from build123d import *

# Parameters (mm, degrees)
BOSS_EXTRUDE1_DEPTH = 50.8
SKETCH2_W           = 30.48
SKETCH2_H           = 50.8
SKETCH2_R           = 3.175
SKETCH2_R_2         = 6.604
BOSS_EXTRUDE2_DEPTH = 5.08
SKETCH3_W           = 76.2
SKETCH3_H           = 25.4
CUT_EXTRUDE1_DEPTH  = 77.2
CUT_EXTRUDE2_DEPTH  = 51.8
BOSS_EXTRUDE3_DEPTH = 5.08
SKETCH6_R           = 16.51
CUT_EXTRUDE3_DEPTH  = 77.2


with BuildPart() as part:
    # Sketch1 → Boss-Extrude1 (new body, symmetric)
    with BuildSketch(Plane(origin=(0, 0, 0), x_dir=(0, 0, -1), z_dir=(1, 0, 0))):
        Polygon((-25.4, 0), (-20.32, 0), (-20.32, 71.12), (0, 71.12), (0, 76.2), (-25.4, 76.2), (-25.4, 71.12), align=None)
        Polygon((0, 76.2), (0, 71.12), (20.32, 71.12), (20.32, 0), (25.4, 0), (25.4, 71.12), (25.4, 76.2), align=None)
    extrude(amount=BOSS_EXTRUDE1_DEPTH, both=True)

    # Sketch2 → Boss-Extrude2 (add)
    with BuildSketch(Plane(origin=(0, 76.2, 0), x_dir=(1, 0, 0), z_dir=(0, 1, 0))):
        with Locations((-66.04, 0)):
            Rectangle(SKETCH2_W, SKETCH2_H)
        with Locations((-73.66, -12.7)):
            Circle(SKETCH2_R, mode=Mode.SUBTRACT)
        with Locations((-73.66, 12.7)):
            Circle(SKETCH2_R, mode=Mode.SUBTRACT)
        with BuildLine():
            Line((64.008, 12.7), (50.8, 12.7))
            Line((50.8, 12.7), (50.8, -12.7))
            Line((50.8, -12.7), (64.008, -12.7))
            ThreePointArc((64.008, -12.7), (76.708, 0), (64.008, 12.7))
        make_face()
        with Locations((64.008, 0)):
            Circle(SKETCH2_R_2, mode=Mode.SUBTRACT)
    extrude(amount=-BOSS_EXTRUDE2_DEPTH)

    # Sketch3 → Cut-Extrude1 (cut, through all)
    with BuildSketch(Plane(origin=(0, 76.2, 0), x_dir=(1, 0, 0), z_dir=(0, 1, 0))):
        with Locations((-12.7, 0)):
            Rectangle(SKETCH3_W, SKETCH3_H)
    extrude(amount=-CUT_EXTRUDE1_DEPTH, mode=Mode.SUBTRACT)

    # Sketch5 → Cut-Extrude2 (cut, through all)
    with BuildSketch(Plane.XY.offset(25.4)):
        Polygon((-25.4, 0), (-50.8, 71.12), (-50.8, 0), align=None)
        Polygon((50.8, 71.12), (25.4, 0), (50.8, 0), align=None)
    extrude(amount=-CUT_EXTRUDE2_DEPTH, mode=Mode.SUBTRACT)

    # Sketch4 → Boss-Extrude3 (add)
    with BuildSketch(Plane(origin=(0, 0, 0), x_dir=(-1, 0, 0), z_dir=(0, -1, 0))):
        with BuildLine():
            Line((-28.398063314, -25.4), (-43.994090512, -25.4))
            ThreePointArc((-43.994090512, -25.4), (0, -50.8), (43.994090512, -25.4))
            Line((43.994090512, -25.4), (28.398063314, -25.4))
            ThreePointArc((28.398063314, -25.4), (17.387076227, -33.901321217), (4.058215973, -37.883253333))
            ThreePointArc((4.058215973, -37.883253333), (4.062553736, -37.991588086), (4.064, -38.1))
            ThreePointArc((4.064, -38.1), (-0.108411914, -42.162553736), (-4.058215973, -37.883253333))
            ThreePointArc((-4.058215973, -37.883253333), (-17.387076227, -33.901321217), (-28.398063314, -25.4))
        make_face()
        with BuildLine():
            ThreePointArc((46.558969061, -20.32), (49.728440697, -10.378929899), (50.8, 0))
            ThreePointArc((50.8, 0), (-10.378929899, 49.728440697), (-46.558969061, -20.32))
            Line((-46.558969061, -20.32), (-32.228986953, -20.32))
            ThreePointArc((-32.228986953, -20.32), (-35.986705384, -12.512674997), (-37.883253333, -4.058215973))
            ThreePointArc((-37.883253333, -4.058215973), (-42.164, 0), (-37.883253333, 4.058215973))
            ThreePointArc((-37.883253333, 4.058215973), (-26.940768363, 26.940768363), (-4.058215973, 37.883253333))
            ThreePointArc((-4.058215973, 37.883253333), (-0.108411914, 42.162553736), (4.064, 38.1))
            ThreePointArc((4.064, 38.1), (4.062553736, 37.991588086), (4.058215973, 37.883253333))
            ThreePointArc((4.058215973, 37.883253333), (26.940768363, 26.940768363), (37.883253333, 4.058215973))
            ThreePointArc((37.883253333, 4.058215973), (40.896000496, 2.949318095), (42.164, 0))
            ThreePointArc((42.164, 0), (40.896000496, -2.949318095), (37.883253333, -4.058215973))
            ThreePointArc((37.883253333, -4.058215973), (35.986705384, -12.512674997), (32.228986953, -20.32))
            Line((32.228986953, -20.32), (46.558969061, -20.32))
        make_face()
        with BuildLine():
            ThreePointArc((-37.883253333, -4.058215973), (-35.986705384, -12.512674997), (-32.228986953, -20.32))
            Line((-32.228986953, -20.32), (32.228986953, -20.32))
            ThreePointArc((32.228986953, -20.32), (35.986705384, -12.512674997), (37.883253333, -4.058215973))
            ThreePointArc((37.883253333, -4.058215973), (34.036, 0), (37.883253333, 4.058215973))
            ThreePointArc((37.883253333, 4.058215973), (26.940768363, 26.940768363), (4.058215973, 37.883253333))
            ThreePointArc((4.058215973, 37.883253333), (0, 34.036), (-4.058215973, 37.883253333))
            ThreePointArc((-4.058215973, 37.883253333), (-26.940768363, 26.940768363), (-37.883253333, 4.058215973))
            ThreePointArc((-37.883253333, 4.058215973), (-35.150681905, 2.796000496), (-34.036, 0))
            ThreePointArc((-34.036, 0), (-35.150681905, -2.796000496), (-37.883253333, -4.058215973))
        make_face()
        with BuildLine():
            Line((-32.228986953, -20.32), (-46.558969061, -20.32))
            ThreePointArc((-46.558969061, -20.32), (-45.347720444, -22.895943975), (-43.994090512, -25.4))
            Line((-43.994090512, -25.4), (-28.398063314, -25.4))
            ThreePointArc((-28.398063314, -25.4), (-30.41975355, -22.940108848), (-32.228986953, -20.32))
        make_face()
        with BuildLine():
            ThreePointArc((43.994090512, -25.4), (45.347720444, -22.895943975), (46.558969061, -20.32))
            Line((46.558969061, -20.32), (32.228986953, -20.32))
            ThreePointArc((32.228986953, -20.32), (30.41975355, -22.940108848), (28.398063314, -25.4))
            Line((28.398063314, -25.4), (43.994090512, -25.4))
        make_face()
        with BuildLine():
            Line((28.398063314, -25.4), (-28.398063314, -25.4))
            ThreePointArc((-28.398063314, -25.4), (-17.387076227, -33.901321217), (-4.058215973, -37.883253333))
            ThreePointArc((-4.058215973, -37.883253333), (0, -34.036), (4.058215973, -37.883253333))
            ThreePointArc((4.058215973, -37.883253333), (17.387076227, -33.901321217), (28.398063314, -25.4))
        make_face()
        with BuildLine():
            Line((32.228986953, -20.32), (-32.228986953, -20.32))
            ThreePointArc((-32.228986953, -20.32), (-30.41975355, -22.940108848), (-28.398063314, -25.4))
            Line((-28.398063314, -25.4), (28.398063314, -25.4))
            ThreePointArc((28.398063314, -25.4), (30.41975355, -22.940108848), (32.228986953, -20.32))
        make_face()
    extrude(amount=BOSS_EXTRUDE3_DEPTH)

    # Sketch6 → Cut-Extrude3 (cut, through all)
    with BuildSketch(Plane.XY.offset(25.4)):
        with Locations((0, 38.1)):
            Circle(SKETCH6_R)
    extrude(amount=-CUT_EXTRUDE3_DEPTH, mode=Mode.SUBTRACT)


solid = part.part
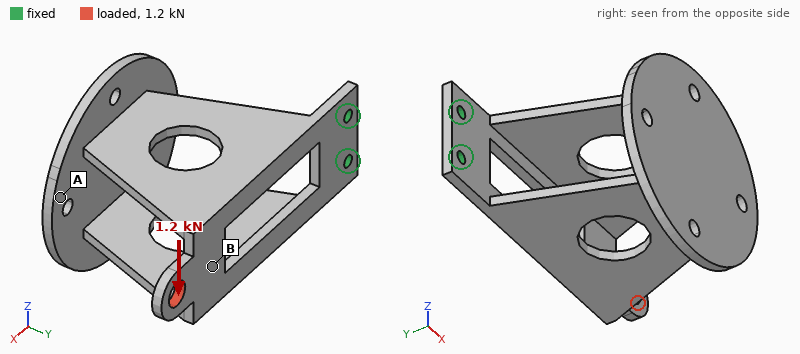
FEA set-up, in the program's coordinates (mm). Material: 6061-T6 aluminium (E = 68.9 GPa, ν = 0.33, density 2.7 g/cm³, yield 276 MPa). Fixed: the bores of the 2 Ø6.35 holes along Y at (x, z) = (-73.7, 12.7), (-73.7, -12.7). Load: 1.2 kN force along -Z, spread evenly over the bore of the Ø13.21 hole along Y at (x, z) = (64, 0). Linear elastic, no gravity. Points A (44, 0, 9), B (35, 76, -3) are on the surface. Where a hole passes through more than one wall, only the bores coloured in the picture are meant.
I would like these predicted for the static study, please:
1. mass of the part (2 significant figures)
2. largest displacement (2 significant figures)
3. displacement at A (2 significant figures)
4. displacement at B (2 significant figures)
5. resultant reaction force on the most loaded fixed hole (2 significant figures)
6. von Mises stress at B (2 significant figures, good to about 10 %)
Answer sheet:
300 g
0.90 mm
0.49 mm
0.73 mm
5.4 kN
40 MPa
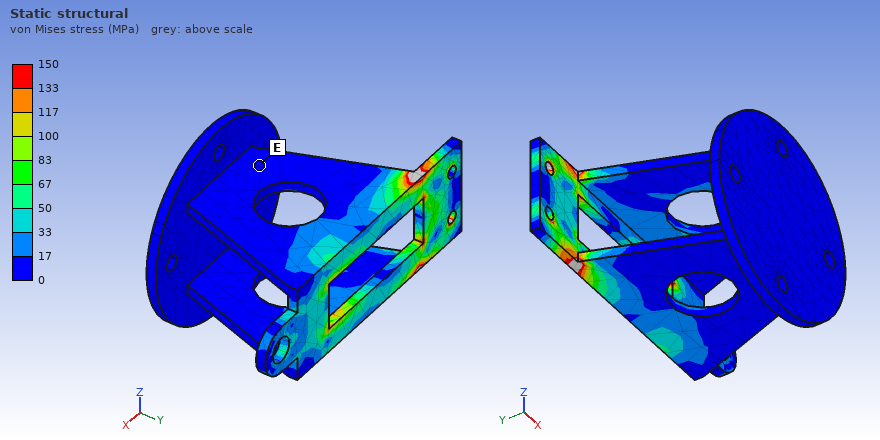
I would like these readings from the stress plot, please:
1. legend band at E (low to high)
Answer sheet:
0 to 17 MPa
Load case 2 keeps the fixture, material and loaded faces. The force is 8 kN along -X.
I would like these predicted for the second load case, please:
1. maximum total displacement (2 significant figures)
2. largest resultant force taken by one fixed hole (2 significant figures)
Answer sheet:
0.29 mm
4.1 kN
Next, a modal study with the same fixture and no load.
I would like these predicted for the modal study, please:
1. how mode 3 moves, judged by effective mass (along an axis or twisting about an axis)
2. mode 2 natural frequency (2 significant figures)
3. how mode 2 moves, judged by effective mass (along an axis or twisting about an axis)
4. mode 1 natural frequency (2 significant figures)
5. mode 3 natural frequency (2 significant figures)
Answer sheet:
along Z
260 Hz
along Z
110 Hz
700 Hz
